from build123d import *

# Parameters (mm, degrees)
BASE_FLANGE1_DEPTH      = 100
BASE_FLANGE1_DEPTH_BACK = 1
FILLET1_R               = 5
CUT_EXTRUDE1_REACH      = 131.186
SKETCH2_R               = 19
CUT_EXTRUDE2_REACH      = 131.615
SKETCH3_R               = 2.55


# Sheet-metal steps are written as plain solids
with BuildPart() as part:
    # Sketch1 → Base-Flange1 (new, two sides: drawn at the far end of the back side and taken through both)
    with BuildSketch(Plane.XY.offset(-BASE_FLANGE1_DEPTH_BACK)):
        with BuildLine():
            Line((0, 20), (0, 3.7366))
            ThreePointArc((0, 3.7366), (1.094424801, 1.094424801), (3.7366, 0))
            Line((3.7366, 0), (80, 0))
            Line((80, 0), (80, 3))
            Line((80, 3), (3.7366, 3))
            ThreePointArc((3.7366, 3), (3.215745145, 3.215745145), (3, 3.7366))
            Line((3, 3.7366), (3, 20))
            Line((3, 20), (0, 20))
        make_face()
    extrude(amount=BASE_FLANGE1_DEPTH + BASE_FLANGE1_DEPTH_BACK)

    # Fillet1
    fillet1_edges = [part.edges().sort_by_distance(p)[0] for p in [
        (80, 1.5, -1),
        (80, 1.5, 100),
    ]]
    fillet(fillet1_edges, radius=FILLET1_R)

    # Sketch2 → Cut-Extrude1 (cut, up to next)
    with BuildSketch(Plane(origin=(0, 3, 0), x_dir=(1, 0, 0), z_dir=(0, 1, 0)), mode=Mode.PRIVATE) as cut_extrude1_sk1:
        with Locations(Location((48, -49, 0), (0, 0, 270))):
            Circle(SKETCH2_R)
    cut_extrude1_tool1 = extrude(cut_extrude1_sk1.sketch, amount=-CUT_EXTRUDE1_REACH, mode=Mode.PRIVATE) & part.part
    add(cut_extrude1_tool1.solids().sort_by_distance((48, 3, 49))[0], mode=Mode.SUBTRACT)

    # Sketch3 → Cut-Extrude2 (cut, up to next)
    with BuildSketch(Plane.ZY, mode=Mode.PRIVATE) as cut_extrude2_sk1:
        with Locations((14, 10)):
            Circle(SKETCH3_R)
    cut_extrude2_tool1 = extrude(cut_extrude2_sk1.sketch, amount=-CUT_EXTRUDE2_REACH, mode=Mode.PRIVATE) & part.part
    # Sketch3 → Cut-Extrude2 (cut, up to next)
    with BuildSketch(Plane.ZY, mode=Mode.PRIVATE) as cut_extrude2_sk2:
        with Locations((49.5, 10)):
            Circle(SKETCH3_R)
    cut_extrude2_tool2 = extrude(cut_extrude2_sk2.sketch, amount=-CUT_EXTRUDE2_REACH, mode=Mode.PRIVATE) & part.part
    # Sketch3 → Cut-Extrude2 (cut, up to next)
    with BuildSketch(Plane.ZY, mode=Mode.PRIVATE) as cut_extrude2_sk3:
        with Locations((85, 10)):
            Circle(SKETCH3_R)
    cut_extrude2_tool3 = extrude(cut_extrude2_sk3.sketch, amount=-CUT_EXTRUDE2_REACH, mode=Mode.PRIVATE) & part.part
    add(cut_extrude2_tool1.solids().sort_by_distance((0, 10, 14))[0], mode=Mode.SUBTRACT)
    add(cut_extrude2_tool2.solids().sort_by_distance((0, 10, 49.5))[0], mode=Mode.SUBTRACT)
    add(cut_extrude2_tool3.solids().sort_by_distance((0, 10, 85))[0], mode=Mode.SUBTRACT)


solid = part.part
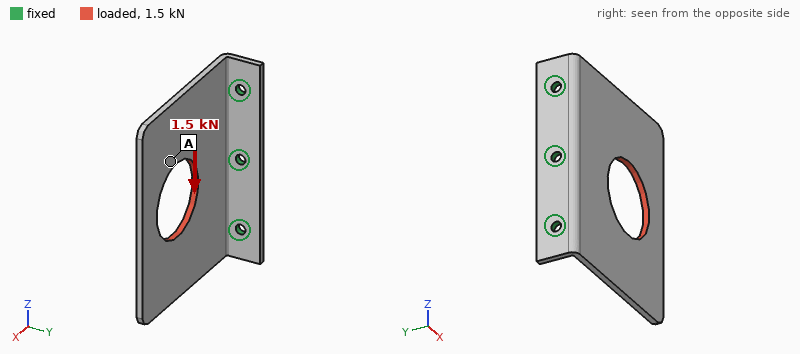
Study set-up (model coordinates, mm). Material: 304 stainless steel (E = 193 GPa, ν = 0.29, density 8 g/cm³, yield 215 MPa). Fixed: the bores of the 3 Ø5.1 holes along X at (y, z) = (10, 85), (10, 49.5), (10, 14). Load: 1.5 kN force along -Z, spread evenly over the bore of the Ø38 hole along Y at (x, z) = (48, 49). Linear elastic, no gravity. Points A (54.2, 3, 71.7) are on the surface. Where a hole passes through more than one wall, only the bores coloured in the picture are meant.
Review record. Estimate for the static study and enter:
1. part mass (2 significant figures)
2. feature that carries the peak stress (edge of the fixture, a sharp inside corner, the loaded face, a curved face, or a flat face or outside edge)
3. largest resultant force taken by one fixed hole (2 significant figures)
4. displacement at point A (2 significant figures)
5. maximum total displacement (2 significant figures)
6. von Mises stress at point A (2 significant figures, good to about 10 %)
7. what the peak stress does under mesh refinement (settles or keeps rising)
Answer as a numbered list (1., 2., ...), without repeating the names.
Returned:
1. 200 g
2. edge of the fixture
3. 1.0 kN
4. 42 µm
5. 81 µm
6. 14 MPa
7. keeps rising
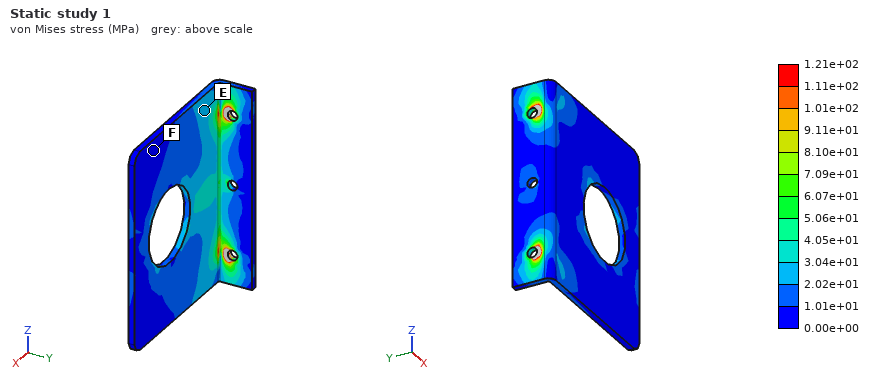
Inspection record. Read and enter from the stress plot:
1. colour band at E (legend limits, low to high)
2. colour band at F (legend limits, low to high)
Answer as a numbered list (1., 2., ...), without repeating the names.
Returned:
1. 2.02e+01 to 3.04e+01 MPa
2. 0.00e+00 to 1.01e+01 MPa
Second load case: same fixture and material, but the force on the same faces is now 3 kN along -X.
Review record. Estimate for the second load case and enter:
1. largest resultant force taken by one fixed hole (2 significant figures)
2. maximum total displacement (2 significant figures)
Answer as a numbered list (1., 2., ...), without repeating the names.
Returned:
1. 1.0 kN
2. 0.21 mm
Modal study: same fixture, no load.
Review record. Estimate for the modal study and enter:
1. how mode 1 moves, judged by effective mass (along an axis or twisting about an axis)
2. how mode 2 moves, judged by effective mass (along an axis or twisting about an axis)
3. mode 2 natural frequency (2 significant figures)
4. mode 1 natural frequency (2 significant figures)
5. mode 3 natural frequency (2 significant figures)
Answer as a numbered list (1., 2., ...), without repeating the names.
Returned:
1. along Y
2. twisting about X
3. 680 Hz
4. 340 Hz
5. 1800 Hz
